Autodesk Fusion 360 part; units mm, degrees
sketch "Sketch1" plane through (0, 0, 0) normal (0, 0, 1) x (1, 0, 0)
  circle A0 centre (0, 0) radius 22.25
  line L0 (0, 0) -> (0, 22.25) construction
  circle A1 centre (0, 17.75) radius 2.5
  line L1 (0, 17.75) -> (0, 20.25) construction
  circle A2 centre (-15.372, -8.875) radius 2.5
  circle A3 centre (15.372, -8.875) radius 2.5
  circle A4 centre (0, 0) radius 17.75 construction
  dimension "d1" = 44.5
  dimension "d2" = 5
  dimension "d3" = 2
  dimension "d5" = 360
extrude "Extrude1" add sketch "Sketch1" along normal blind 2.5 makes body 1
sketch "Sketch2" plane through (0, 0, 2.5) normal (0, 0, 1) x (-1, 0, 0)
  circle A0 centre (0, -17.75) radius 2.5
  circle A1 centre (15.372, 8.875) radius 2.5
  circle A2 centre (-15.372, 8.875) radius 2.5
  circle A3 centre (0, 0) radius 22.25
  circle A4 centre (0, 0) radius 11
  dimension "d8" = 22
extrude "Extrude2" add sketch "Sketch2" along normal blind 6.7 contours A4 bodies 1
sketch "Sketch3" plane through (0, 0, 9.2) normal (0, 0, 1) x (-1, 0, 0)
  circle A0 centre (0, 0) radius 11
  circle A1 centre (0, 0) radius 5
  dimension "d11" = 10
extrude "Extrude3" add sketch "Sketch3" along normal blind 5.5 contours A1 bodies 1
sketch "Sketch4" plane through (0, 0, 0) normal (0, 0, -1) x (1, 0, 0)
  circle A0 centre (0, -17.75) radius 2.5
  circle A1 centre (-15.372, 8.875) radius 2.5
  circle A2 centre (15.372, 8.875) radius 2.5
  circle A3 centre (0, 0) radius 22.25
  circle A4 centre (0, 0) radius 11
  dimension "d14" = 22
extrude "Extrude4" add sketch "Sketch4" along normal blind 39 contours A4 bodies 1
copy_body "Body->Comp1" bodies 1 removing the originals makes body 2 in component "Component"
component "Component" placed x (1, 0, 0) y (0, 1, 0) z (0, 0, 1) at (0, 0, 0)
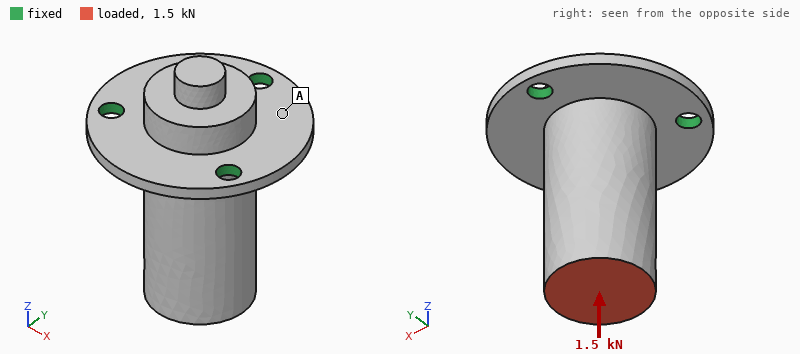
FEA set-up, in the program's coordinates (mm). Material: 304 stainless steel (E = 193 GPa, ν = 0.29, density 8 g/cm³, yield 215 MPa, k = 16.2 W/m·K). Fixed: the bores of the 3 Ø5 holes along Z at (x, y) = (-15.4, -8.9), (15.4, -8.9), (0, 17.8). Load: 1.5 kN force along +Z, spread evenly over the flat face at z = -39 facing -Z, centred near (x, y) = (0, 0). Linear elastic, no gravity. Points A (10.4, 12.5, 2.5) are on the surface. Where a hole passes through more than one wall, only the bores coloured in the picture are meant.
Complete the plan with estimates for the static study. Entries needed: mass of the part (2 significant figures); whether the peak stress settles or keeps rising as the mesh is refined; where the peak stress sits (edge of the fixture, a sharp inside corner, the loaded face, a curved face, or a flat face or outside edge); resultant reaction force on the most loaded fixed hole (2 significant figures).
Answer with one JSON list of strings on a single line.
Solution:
["170 g", "keeps rising", "edge of the fixture", "500 N"]
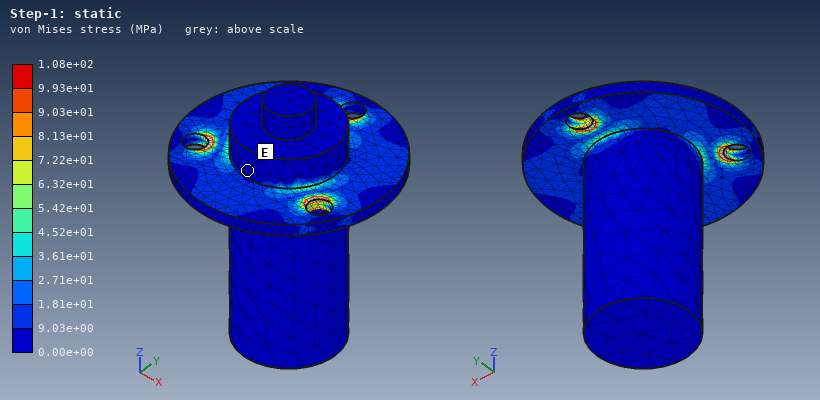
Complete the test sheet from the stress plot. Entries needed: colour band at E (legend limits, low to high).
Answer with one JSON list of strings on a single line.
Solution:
["0.00e+00 to 9.03e+00 MPa"]
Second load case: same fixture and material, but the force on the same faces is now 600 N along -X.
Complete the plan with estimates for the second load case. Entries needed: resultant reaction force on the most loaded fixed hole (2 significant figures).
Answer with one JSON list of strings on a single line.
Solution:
["950 N"]
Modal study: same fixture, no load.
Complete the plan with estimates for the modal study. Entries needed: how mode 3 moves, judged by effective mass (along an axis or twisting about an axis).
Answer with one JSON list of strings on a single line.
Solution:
["along Z"]
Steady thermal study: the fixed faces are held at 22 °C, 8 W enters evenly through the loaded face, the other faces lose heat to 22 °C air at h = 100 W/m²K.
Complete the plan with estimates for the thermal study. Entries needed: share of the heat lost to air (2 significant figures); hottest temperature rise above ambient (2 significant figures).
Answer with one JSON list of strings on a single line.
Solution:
["80 %", "38 K"]
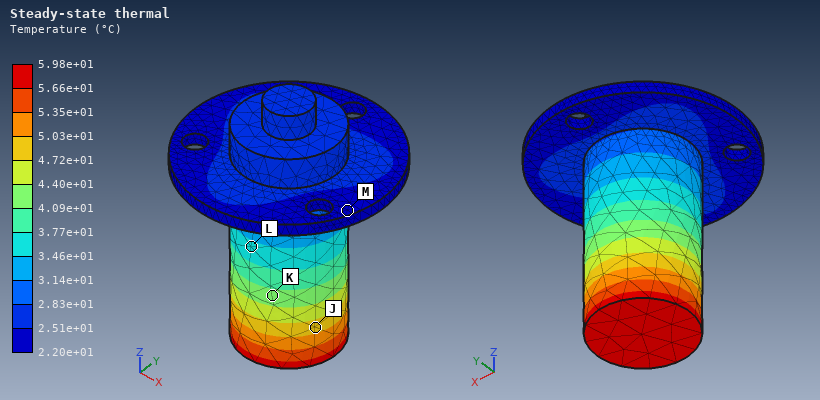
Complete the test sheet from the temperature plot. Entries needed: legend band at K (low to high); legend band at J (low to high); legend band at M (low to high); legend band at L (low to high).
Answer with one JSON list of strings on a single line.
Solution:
["4.09e+01 to 4.40e+01 °C", "4.72e+01 to 5.03e+01 °C", "2.20e+01 to 2.51e+01 °C", "3.46e+01 to 3.77e+01 °C"]
